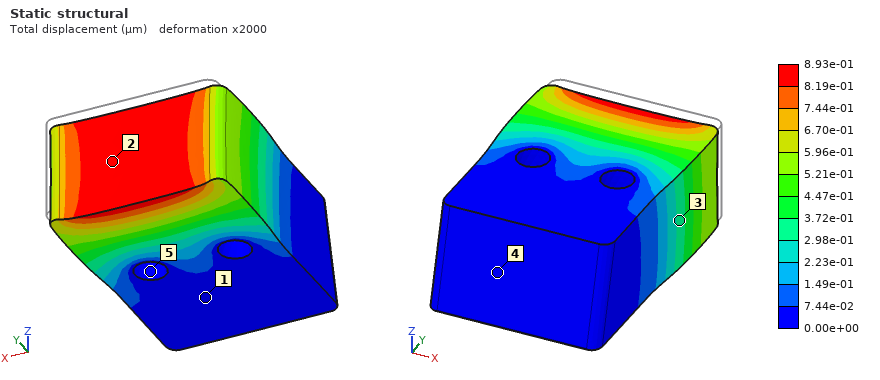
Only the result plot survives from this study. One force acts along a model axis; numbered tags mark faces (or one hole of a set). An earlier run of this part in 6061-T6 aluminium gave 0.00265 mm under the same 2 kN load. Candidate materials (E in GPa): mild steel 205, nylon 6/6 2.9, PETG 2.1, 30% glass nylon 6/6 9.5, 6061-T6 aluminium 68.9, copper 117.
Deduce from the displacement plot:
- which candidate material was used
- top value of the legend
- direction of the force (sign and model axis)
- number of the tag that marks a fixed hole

mild steel
8.93e-01 µm
-Y
5
